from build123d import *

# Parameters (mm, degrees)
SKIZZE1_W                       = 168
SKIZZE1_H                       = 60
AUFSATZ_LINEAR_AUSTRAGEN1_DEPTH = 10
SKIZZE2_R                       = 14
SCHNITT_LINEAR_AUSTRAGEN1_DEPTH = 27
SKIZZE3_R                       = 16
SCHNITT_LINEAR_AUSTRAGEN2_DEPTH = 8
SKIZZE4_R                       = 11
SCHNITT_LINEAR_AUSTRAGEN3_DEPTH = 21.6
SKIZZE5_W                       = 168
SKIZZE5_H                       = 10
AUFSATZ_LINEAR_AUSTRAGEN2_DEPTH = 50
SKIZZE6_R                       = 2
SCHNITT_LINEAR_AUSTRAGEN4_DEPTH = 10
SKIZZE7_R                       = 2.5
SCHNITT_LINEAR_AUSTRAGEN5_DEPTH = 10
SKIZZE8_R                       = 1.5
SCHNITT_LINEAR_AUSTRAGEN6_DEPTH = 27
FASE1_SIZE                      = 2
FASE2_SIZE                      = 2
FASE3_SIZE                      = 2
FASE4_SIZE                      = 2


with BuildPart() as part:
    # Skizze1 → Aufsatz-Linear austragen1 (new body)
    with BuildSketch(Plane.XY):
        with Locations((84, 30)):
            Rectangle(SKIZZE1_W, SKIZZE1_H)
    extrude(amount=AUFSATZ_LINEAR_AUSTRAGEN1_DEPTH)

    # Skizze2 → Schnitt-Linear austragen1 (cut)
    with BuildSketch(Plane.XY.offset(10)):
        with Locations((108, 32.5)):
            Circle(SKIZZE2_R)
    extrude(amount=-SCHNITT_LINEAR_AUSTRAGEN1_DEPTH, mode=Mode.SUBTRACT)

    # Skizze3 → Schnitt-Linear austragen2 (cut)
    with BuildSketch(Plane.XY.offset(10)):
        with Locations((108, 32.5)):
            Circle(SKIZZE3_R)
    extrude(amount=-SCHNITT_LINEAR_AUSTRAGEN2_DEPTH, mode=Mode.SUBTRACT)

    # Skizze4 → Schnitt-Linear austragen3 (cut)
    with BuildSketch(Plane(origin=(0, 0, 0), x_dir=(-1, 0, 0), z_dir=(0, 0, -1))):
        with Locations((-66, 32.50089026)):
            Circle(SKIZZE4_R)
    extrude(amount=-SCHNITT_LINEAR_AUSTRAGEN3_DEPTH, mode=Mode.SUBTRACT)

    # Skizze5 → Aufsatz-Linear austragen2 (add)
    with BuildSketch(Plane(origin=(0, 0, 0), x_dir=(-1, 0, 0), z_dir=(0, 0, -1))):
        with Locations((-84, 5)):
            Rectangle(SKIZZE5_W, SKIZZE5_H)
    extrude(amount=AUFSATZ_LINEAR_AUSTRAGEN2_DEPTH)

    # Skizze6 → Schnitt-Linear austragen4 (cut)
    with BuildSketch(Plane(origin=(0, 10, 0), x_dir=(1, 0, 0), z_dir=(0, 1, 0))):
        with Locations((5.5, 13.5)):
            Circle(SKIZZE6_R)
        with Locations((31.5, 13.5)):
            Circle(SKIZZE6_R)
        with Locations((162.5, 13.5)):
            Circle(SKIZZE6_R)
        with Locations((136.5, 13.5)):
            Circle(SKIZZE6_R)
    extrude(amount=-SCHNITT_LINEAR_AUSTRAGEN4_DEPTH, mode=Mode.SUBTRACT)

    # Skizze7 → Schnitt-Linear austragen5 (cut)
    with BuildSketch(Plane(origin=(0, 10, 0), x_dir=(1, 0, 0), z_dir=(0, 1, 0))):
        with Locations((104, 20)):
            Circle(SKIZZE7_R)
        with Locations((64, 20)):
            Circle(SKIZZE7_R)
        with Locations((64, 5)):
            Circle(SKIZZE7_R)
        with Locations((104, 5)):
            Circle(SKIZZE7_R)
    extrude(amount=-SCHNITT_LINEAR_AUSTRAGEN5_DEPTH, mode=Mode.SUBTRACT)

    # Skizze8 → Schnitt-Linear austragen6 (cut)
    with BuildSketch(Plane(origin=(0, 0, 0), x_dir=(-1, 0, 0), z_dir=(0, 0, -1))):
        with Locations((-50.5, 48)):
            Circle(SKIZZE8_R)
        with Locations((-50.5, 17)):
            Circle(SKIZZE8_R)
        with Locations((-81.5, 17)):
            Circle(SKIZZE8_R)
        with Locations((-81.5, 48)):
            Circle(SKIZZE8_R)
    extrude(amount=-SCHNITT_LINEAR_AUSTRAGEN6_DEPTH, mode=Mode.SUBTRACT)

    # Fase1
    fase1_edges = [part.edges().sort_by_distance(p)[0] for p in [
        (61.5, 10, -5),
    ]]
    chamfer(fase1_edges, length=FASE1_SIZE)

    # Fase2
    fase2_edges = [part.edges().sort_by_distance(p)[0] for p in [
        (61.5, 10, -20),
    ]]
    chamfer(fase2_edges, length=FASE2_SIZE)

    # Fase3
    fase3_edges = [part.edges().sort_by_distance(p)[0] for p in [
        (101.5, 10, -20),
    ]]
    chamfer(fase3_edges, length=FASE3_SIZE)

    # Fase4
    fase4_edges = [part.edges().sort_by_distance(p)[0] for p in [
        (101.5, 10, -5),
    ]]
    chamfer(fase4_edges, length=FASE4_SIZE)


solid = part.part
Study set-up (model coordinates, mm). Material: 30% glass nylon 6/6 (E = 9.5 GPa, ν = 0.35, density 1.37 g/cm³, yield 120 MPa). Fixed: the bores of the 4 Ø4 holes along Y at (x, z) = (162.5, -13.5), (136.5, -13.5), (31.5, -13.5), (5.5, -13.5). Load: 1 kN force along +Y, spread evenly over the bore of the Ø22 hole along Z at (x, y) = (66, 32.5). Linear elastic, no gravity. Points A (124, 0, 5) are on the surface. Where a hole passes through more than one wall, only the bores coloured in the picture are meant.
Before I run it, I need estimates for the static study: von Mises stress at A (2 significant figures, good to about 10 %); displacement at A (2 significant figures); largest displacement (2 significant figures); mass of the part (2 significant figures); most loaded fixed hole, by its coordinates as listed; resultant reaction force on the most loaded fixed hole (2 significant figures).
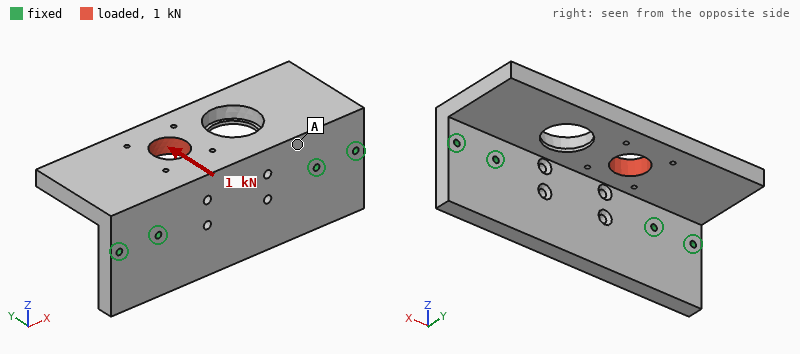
1.8 MPa
0.046 mm
0.19 mm
240 g
(31.5, -13.5)
520 N
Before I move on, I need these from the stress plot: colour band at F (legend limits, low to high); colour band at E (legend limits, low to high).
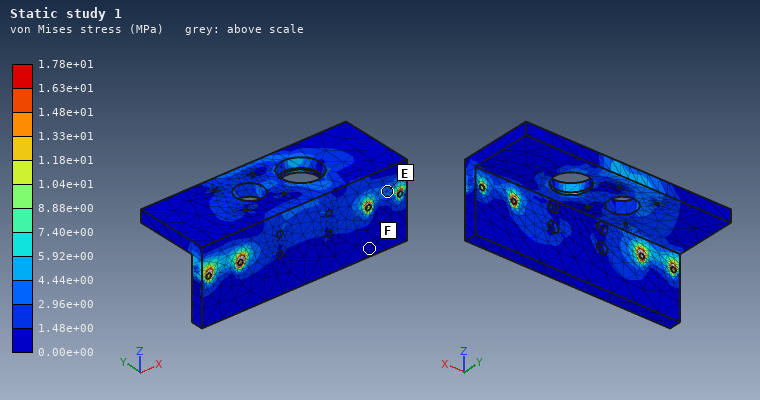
0.00e+00 to 1.48e+00 MPa
2.96e+00 to 4.44e+00 MPa
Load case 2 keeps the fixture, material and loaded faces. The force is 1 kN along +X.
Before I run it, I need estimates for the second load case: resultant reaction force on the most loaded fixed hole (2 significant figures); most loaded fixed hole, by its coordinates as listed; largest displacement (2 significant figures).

380 N
(31.5, -13.5)
53 µm
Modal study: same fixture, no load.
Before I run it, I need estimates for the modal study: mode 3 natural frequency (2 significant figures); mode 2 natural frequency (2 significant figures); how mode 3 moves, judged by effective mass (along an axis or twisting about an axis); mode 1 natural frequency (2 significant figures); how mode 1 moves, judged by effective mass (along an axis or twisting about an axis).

1800 Hz
1200 Hz
along Y
790 Hz
along Z
